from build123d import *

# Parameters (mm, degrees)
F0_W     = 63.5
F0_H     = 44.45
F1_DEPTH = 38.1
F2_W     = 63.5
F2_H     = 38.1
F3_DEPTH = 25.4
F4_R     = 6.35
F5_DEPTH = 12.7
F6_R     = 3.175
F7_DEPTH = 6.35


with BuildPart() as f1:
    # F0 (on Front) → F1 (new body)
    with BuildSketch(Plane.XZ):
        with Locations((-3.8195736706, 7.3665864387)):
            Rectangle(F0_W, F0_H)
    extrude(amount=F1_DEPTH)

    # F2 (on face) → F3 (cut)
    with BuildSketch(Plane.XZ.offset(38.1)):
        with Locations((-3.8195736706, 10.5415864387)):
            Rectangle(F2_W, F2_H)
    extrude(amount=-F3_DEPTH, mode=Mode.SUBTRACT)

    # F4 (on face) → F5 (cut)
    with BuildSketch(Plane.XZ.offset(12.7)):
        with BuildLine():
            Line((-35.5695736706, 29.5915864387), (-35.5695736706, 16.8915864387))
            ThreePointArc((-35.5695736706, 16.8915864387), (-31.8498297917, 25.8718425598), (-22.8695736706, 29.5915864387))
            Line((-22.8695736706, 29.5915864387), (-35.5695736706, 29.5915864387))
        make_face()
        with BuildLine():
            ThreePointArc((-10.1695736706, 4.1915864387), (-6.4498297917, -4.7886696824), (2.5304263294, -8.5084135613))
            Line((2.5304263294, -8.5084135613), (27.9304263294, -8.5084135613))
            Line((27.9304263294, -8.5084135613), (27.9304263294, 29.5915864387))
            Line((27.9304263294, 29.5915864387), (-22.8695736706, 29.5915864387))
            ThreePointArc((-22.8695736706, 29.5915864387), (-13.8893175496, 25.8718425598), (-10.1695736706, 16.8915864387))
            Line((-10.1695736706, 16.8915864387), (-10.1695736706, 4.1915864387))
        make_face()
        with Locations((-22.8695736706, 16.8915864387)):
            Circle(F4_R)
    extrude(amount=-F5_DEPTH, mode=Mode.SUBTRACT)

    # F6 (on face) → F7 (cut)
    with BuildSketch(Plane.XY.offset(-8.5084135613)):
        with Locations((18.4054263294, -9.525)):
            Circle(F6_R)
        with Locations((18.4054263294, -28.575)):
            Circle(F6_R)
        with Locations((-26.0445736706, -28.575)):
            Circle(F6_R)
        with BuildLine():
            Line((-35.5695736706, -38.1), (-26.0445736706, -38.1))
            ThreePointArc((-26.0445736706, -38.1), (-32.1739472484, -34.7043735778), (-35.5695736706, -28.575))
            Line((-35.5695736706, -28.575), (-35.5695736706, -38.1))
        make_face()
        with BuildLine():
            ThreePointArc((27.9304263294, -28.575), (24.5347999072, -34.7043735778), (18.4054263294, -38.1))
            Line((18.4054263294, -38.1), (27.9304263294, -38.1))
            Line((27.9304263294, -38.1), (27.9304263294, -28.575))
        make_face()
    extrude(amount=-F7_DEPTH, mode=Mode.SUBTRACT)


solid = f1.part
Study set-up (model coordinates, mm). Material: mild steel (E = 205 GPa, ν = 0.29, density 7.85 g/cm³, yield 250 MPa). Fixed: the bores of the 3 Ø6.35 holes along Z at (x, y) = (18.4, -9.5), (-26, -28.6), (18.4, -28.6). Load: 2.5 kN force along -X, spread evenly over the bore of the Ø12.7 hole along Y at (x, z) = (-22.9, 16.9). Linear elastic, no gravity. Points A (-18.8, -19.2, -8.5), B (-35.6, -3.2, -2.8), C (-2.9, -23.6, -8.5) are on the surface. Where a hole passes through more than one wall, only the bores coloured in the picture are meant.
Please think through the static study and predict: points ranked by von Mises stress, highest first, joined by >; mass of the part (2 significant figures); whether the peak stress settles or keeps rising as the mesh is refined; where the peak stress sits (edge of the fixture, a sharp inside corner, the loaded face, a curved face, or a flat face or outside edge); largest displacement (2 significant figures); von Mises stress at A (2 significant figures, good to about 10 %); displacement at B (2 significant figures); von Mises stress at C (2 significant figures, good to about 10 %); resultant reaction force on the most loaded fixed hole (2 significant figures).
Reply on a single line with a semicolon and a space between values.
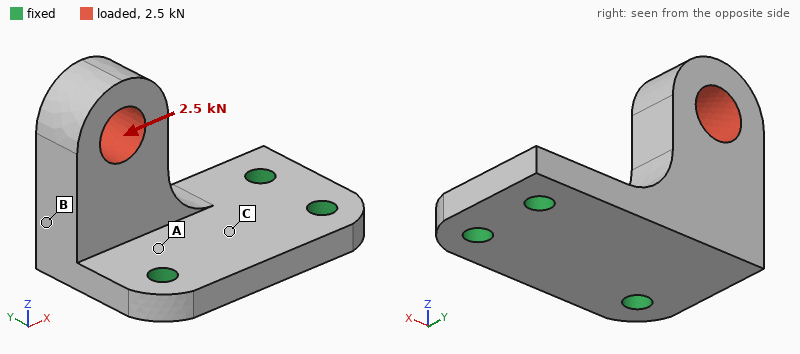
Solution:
A > C > B; 190 g; keeps rising; edge of the fixture; 94 µm; 83 MPa; 51 µm; 38 MPa; 1.9 kN
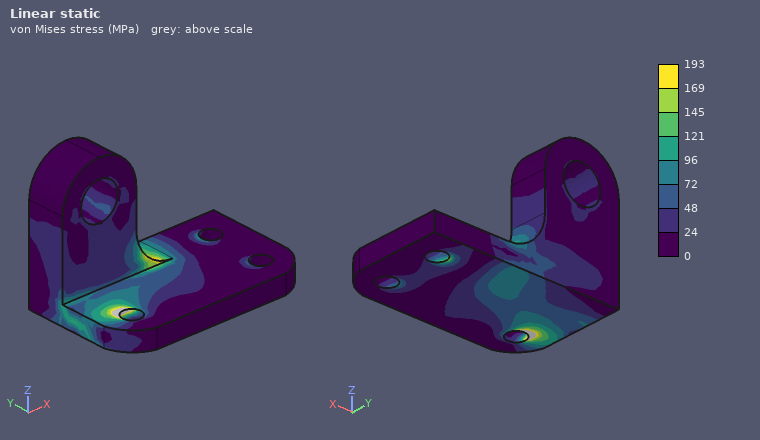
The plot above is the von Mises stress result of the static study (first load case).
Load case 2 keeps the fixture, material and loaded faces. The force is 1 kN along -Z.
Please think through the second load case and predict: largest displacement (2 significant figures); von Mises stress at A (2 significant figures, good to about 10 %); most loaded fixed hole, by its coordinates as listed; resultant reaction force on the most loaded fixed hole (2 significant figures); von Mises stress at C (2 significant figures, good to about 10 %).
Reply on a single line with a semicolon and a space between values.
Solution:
42 µm; 30 MPa; (-26, -28.6); 810 N; 16 MPa
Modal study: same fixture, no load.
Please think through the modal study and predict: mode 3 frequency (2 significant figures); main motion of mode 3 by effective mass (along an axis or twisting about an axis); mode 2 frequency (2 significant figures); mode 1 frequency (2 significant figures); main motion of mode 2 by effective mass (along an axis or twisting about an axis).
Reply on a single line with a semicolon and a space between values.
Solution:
7700 Hz; along Z; 5100 Hz; 2400 Hz; along X
